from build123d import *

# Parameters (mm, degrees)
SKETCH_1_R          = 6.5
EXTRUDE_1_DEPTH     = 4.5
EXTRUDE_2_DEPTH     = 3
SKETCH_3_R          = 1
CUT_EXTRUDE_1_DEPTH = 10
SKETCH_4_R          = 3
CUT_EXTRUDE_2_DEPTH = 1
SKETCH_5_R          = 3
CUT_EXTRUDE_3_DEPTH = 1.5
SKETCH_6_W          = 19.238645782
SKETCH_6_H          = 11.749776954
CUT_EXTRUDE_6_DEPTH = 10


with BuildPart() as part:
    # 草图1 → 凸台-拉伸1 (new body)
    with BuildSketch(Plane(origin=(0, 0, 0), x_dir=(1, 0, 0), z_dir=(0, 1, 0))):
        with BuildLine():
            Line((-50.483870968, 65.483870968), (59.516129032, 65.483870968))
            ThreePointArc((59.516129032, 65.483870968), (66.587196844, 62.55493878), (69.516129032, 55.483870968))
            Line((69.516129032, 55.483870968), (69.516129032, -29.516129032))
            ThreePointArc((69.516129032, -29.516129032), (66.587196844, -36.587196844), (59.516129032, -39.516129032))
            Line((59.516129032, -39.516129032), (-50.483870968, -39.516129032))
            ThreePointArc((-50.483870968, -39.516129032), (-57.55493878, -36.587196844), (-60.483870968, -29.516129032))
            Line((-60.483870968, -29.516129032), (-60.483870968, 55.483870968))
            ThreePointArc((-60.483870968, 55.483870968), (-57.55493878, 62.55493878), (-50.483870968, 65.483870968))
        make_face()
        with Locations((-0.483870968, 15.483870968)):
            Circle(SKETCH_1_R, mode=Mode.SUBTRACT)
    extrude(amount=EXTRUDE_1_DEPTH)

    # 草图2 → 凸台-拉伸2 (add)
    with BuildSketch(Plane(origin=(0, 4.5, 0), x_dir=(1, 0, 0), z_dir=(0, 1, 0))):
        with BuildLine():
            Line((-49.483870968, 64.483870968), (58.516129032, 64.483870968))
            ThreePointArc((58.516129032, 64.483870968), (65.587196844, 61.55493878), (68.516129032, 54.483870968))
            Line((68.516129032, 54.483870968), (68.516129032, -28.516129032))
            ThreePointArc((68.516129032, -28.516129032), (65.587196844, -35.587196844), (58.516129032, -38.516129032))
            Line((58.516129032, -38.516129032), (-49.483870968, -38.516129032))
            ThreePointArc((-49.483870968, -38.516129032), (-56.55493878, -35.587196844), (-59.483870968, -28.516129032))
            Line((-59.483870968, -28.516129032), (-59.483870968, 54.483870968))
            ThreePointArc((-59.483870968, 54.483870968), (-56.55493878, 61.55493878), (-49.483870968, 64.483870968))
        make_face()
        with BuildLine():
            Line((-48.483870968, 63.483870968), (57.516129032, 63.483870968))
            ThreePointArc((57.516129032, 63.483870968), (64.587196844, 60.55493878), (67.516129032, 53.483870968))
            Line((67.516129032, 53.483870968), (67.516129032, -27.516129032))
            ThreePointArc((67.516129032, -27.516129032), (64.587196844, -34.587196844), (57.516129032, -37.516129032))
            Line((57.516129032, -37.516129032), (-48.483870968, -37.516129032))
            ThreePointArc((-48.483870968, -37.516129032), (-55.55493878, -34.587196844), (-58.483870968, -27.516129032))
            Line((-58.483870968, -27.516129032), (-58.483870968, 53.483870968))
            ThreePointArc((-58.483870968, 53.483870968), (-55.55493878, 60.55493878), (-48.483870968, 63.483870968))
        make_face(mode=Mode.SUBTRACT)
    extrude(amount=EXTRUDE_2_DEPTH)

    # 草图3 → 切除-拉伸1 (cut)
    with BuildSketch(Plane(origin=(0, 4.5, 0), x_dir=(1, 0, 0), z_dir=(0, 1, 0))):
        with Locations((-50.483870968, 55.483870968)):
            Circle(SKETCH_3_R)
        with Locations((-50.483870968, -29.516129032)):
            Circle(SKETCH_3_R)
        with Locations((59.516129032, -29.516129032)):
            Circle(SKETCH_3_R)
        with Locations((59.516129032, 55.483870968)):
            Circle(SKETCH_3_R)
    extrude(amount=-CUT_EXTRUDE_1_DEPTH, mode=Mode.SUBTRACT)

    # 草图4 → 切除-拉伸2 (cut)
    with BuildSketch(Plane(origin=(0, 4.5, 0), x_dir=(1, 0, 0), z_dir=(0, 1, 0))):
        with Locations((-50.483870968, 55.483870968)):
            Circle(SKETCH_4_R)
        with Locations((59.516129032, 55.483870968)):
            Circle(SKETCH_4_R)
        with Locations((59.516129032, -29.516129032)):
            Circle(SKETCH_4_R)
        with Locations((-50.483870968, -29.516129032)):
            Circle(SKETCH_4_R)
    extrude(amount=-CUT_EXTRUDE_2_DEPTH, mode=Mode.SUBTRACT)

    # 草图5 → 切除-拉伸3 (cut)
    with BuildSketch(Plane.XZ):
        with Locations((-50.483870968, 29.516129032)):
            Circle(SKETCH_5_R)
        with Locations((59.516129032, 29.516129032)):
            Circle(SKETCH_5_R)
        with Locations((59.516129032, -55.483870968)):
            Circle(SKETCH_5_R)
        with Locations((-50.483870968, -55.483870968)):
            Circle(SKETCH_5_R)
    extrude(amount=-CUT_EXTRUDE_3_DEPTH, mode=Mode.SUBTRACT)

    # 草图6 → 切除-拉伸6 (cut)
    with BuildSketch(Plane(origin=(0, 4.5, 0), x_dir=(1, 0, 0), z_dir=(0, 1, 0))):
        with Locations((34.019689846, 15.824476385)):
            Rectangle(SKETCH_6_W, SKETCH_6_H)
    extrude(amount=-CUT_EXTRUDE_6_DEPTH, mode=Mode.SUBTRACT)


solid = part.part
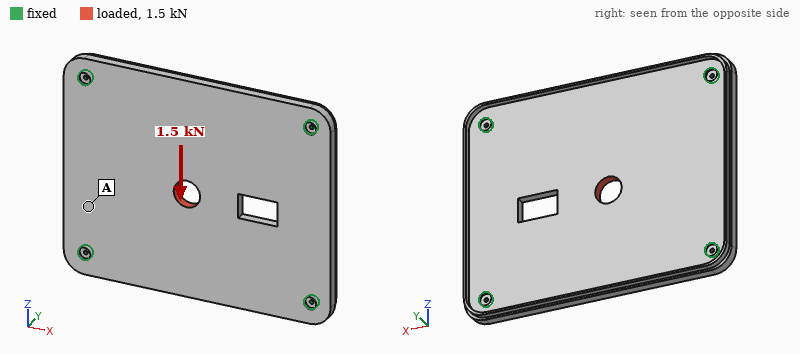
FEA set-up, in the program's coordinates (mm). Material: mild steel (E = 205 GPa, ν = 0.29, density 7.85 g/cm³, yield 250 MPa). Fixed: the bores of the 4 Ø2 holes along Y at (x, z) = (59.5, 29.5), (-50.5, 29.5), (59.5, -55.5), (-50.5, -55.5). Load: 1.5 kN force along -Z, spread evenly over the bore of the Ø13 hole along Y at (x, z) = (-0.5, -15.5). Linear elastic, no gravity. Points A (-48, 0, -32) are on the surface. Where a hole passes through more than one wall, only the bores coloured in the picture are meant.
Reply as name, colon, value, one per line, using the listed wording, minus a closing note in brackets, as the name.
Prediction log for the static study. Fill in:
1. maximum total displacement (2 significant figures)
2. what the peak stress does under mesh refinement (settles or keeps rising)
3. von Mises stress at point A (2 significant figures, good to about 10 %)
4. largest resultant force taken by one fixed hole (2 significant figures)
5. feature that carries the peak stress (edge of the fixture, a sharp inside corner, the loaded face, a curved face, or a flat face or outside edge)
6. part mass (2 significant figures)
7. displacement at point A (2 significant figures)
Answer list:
maximum total displacement: 2.4 µm
what the peak stress does under mesh refinement: keeps rising
von Mises stress at point A: 2.4 MPa
largest resultant force taken by one fixed hole: 470 N
feature that carries the peak stress: edge of the fixture
part mass: 470 g
displacement at point A: 0.74 µm
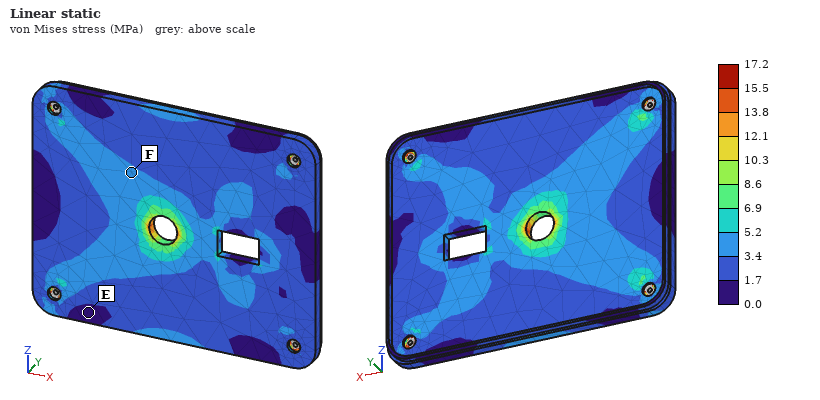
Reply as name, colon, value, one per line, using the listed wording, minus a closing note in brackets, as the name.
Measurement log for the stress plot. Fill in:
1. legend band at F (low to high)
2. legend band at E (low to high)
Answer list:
legend band at F: 3.4 to 5.2 MPa
legend band at E: 0.0 to 1.7 MPa
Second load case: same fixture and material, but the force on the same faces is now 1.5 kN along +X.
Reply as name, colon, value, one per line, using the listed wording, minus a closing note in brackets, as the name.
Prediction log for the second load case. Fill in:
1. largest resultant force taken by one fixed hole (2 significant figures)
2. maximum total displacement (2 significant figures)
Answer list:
largest resultant force taken by one fixed hole: 410 N
maximum total displacement: 1.9 µm
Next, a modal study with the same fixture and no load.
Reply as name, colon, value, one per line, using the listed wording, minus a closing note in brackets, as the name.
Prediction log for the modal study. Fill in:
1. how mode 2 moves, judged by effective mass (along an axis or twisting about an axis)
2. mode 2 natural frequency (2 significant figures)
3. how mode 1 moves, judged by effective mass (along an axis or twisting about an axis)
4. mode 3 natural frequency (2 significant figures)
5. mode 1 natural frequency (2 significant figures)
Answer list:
how mode 2 moves, judged by effective mass: twisting about X
mode 2 natural frequency: 1800 Hz
how mode 1 moves, judged by effective mass: along Y
mode 3 natural frequency: 2100 Hz
mode 1 natural frequency: 1100 Hz
